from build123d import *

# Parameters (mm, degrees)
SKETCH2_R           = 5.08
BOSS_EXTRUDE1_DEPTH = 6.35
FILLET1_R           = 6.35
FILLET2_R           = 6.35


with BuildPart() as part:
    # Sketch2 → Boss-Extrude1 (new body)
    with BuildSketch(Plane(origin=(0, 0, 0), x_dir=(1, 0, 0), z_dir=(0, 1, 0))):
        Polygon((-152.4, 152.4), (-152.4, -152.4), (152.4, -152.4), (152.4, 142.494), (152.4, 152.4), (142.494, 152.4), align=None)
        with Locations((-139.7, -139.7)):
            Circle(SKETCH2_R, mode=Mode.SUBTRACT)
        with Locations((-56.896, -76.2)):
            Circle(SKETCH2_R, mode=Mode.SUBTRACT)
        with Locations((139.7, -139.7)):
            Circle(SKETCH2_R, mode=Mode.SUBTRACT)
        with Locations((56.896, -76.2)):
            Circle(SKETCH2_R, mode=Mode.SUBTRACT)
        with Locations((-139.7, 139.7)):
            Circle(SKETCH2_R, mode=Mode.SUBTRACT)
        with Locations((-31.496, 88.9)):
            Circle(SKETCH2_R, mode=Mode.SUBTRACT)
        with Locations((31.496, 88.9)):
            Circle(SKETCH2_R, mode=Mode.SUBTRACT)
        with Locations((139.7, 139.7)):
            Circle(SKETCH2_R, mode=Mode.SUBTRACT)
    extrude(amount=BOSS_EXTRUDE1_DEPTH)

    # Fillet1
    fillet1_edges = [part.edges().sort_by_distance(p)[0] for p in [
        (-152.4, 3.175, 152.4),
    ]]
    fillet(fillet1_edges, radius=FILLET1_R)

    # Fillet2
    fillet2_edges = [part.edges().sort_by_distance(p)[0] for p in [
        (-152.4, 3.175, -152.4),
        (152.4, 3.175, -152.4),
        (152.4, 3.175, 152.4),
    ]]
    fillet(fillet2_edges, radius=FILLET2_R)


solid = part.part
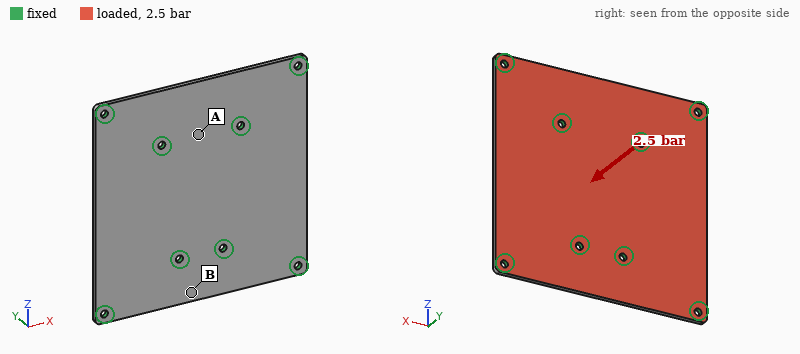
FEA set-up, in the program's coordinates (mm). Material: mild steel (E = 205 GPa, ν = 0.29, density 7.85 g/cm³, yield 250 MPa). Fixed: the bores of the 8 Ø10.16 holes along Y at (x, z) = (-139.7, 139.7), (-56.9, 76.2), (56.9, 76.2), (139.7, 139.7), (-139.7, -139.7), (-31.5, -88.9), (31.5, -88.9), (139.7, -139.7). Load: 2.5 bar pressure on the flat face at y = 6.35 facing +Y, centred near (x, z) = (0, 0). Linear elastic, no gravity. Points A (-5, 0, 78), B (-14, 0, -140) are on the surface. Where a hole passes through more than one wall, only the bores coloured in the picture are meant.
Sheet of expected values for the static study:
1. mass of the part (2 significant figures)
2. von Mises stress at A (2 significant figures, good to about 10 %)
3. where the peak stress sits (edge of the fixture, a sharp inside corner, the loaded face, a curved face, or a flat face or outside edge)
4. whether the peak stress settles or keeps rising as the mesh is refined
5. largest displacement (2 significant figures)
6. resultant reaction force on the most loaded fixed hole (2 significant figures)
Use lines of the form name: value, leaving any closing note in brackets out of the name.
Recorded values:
mass of the part: 4.6 kg
von Mises stress at A: 43 MPa
where the peak stress sits: edge of the fixture
whether the peak stress settles or keeps rising as the mesh is refined: keeps rising
largest displacement: 0.52 mm
resultant reaction force on the most loaded fixed hole: 4.7 kN
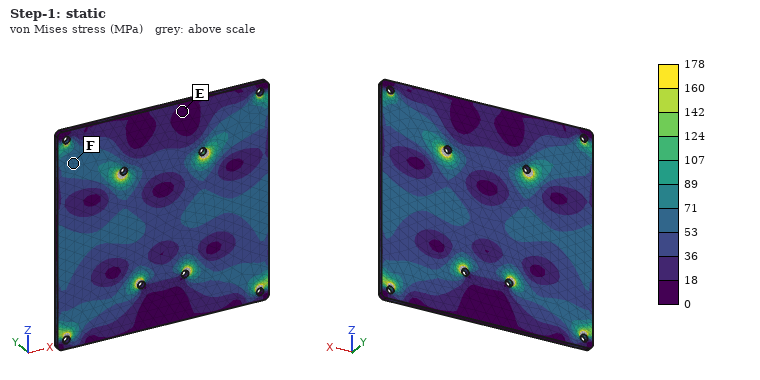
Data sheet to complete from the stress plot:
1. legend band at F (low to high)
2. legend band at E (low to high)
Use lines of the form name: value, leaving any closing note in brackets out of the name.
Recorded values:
legend band at F: 53 to 71 MPa
legend band at E: 0 to 18 MPa
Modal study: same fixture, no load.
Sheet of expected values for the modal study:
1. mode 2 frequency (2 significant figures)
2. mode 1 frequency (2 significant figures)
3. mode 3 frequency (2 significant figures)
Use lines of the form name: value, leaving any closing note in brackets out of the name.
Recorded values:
mode 2 frequency: 640 Hz
mode 1 frequency: 640 Hz
mode 3 frequency: 1000 Hz
